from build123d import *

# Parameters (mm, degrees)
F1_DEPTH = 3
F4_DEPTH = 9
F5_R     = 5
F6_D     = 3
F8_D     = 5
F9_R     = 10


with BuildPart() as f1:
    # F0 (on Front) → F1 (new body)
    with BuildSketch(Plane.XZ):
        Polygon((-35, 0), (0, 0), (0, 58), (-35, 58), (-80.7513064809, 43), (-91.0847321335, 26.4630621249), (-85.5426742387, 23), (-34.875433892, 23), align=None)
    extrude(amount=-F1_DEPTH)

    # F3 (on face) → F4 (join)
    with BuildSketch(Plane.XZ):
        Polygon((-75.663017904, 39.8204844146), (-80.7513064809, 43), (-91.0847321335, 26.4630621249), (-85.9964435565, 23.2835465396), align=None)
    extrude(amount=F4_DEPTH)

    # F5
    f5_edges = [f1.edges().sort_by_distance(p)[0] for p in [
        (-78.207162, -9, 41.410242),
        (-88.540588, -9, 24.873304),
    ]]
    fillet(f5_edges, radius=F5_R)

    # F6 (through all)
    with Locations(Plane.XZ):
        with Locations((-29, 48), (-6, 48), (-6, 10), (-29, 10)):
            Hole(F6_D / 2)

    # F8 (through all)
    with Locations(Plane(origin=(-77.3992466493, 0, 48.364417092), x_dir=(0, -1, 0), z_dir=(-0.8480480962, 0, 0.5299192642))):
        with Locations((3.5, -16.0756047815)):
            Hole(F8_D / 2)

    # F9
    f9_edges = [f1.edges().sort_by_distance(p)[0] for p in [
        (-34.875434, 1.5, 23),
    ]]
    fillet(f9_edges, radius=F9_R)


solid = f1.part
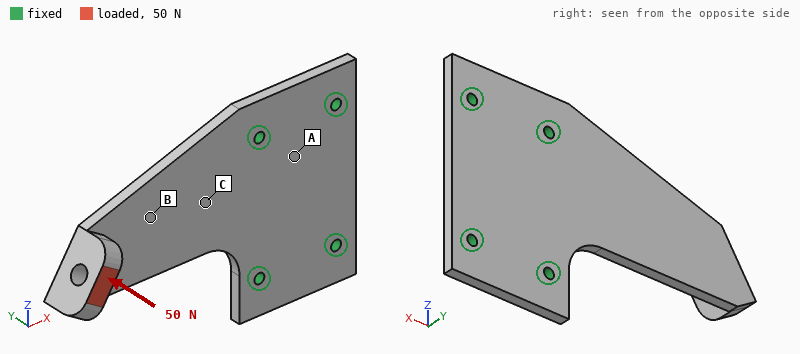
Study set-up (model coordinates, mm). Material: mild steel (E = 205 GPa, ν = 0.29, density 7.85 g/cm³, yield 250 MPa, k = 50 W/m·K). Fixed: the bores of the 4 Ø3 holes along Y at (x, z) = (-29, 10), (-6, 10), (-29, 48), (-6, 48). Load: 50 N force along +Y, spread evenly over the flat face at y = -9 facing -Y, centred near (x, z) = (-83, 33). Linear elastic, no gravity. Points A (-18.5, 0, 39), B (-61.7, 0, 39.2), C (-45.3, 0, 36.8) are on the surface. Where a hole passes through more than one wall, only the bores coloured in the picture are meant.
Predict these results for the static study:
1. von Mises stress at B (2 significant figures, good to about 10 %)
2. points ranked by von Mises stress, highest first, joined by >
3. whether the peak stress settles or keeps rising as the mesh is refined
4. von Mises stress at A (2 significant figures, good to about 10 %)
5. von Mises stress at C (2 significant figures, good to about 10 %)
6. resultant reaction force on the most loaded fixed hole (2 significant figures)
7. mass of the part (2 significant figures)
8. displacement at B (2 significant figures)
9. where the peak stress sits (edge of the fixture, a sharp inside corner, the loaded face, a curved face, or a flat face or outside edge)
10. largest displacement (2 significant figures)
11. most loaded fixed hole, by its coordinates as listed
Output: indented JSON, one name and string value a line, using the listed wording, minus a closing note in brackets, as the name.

{
  "von Mises stress at B": "29 MPa",
  "points ranked by von Mises stress, highest first, joined by >": "C > B > A",
  "whether the peak stress settles or keeps rising as the mesh is refined": "keeps rising",
  "von Mises stress at A": "6.6 MPa",
  "von Mises stress at C": "39 MPa",
  "resultant reaction force on the most loaded fixed hole": "71 N",
  "mass of the part": "87 g",
  "displacement at B": "0.082 mm",
  "where the peak stress sits": "edge of the fixture",
  "largest displacement": "0.24 mm",
  "most loaded fixed hole, by its coordinates as listed": "(-29, 48)"
}
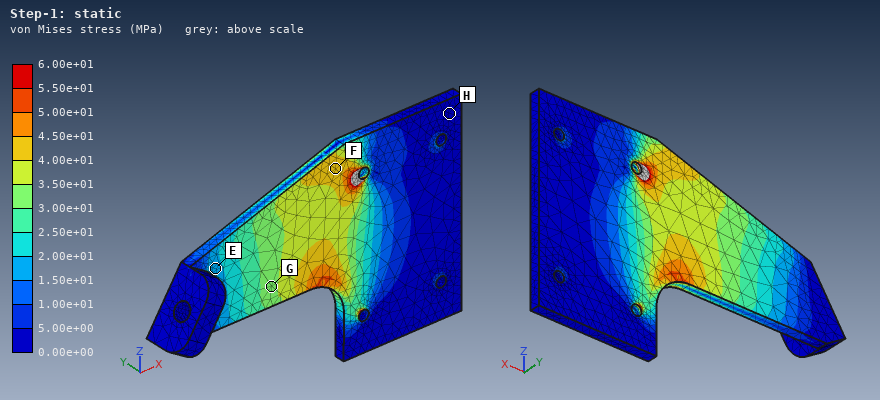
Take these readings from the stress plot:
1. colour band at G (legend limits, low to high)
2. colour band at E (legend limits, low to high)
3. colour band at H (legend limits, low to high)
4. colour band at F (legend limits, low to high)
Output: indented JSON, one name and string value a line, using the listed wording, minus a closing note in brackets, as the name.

{
  "colour band at G": "3.00e+01 to 3.50e+01 MPa",
  "colour band at E": "1.50e+01 to 2.00e+01 MPa",
  "colour band at H": "0.00e+00 to 5.00e+00 MPa",
  "colour band at F": "4.00e+01 to 4.50e+01 MPa"
}
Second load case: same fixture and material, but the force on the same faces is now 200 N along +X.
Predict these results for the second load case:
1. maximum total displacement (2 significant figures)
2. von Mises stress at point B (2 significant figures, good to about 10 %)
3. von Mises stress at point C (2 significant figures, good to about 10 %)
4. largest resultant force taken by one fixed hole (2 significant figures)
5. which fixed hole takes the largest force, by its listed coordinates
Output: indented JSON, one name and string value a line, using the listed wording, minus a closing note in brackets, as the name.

{
  "maximum total displacement": "0.30 mm",
  "von Mises stress at point B": "55 MPa",
  "von Mises stress at point C": "45 MPa",
  "largest resultant force taken by one fixed hole": "93 N",
  "which fixed hole takes the largest force, by its listed coordinates": "(-29, 48)"
}
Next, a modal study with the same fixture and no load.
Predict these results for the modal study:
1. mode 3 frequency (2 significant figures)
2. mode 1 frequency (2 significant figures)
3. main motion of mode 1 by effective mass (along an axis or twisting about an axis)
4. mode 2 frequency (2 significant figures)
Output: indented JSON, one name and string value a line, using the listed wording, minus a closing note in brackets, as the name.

{
  "mode 3 frequency": "3700 Hz",
  "mode 1 frequency": "640 Hz",
  "main motion of mode 1 by effective mass": "along Y",
  "mode 2 frequency": "3300 Hz"
}
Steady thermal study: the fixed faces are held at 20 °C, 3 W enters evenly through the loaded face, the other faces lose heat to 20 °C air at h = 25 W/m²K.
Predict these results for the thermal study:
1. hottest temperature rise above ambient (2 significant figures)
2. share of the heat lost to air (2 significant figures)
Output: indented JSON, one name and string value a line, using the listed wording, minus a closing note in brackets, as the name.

{
  "hottest temperature rise above ambient": "35 K",
  "share of the heat lost to air": "48 %"
}
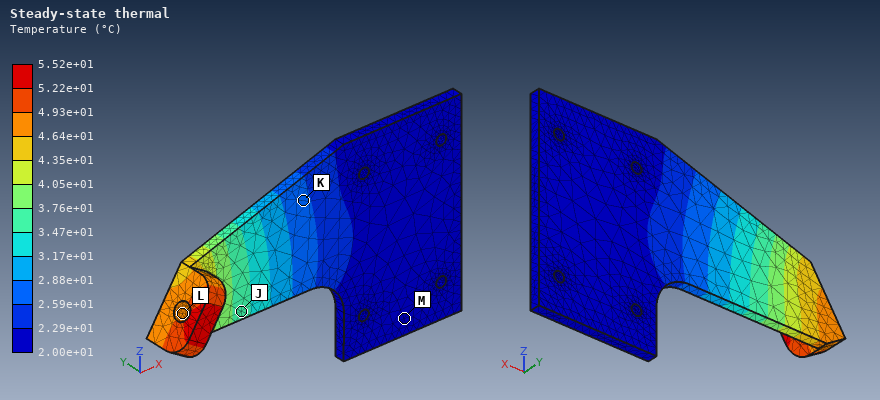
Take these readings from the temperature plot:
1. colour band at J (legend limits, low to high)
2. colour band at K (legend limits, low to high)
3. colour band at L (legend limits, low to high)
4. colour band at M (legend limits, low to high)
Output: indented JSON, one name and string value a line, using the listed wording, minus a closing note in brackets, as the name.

{
  "colour band at J": "3.47e+01 to 3.76e+01 °C",
  "colour band at K": "2.59e+01 to 2.88e+01 °C",
  "colour band at L": "4.64e+01 to 4.93e+01 °C",
  "colour band at M": "2.00e+01 to 2.29e+01 °C"
}
